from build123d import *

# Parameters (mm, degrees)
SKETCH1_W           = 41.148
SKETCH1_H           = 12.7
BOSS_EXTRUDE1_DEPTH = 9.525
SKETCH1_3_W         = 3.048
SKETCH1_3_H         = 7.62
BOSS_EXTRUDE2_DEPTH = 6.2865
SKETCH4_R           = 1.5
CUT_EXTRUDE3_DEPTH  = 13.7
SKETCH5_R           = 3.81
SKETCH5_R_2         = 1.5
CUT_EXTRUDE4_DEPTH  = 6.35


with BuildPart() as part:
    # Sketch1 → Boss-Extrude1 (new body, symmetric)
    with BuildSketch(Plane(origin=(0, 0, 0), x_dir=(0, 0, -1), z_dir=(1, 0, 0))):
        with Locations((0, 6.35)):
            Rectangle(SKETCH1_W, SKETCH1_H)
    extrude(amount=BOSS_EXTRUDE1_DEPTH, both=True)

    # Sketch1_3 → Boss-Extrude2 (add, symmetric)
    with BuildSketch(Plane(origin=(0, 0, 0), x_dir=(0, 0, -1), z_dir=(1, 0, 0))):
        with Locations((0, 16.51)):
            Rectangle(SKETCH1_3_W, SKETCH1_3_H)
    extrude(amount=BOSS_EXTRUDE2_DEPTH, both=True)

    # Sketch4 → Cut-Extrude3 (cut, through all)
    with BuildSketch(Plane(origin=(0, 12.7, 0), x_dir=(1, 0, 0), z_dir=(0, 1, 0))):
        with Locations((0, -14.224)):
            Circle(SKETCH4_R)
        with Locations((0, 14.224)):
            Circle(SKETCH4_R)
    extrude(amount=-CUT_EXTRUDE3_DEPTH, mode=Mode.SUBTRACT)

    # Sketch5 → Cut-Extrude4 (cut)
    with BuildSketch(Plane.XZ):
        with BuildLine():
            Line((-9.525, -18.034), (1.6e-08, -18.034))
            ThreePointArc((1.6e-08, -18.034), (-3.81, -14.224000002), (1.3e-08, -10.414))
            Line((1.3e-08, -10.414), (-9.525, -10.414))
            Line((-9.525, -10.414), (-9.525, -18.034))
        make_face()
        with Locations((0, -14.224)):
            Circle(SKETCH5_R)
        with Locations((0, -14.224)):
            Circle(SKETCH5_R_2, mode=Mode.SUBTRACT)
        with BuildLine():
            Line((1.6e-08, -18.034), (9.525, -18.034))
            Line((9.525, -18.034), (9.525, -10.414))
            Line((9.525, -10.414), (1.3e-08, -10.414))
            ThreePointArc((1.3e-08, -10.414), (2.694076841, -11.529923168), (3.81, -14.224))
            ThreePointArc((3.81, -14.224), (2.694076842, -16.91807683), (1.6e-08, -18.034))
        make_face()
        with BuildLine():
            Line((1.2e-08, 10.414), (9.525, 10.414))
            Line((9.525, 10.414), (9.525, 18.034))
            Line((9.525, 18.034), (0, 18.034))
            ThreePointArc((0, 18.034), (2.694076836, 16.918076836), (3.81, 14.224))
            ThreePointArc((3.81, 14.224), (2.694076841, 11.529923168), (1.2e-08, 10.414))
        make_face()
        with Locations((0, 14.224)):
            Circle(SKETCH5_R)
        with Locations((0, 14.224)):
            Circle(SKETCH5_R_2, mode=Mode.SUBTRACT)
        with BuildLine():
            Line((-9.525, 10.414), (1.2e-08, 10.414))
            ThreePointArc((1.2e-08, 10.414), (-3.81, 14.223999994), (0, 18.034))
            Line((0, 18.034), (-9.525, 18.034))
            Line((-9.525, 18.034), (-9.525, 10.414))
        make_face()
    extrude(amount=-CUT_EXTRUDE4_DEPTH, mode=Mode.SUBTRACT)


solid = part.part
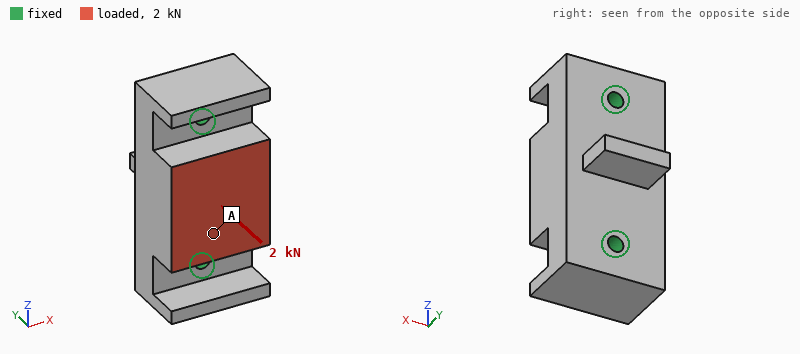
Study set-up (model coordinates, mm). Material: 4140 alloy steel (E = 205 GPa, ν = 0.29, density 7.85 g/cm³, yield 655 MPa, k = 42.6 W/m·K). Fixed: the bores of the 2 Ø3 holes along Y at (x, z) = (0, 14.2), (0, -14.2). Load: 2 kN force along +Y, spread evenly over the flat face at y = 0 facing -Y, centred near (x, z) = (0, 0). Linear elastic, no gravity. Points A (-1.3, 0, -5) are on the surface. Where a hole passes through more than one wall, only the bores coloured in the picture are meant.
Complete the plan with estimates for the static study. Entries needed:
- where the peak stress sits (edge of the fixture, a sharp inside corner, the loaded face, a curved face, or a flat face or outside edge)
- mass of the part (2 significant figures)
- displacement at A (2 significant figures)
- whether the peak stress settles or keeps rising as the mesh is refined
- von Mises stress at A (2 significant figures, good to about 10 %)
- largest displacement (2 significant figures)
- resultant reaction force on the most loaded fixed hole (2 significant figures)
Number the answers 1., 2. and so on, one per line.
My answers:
1. edge of the fixture
2. 65 g
3. 1.8 µm
4. keeps rising
5. 8.4 MPa
6. 2.1 µm
7. 1.1 kN
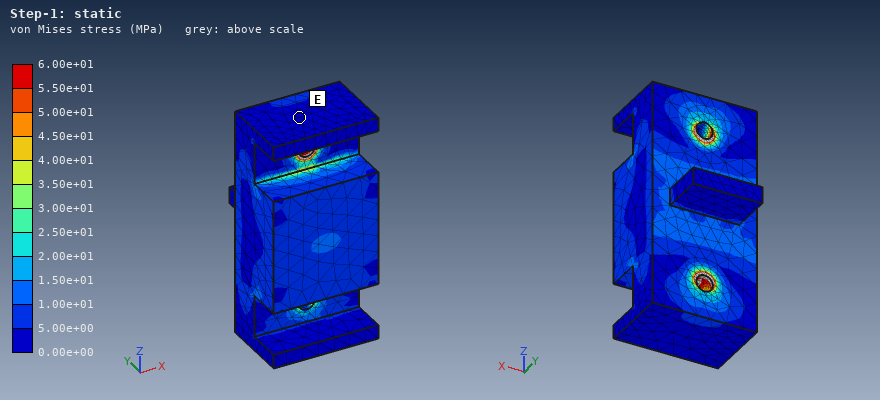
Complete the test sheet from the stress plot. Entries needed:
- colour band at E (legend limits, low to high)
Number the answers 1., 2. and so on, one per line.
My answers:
1. 0.00e+00 to 5.00e+00 MPa
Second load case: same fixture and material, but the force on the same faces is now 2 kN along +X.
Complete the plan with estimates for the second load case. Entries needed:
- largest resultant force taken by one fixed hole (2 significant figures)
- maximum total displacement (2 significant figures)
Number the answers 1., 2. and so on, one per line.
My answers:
1. 1.0 kN
2. 11 µm
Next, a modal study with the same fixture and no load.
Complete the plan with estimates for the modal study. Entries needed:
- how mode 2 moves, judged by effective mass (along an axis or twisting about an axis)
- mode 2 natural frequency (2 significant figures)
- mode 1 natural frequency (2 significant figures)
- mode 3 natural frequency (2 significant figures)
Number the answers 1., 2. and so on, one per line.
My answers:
1. along Y
2. 25 kHz
3. 16 kHz
4. 29 kHz
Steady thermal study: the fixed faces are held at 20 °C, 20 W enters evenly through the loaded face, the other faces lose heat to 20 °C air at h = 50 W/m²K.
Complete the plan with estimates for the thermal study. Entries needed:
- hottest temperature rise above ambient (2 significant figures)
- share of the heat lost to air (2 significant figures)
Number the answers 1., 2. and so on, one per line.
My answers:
1. 25 K
2. 8.2 %
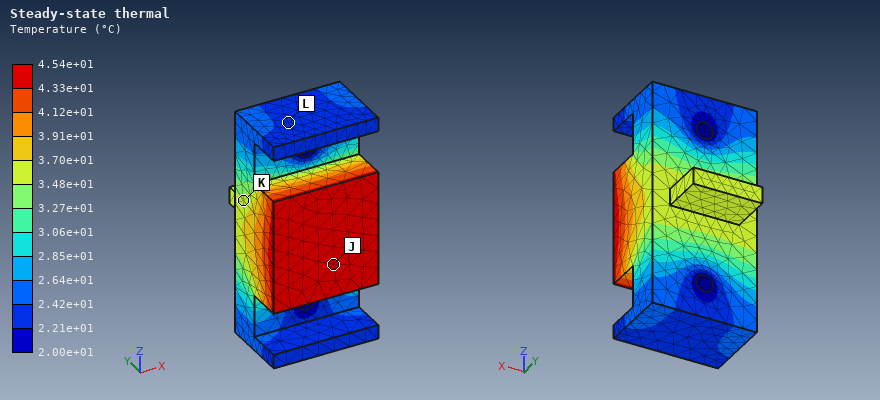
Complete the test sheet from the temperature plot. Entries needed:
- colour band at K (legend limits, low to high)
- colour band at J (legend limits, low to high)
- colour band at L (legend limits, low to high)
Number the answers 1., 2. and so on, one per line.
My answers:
1. 3.48e+01 to 3.70e+01 °C
2. 4.33e+01 to 4.54e+01 °C
3. 2.21e+01 to 2.42e+01 °C
